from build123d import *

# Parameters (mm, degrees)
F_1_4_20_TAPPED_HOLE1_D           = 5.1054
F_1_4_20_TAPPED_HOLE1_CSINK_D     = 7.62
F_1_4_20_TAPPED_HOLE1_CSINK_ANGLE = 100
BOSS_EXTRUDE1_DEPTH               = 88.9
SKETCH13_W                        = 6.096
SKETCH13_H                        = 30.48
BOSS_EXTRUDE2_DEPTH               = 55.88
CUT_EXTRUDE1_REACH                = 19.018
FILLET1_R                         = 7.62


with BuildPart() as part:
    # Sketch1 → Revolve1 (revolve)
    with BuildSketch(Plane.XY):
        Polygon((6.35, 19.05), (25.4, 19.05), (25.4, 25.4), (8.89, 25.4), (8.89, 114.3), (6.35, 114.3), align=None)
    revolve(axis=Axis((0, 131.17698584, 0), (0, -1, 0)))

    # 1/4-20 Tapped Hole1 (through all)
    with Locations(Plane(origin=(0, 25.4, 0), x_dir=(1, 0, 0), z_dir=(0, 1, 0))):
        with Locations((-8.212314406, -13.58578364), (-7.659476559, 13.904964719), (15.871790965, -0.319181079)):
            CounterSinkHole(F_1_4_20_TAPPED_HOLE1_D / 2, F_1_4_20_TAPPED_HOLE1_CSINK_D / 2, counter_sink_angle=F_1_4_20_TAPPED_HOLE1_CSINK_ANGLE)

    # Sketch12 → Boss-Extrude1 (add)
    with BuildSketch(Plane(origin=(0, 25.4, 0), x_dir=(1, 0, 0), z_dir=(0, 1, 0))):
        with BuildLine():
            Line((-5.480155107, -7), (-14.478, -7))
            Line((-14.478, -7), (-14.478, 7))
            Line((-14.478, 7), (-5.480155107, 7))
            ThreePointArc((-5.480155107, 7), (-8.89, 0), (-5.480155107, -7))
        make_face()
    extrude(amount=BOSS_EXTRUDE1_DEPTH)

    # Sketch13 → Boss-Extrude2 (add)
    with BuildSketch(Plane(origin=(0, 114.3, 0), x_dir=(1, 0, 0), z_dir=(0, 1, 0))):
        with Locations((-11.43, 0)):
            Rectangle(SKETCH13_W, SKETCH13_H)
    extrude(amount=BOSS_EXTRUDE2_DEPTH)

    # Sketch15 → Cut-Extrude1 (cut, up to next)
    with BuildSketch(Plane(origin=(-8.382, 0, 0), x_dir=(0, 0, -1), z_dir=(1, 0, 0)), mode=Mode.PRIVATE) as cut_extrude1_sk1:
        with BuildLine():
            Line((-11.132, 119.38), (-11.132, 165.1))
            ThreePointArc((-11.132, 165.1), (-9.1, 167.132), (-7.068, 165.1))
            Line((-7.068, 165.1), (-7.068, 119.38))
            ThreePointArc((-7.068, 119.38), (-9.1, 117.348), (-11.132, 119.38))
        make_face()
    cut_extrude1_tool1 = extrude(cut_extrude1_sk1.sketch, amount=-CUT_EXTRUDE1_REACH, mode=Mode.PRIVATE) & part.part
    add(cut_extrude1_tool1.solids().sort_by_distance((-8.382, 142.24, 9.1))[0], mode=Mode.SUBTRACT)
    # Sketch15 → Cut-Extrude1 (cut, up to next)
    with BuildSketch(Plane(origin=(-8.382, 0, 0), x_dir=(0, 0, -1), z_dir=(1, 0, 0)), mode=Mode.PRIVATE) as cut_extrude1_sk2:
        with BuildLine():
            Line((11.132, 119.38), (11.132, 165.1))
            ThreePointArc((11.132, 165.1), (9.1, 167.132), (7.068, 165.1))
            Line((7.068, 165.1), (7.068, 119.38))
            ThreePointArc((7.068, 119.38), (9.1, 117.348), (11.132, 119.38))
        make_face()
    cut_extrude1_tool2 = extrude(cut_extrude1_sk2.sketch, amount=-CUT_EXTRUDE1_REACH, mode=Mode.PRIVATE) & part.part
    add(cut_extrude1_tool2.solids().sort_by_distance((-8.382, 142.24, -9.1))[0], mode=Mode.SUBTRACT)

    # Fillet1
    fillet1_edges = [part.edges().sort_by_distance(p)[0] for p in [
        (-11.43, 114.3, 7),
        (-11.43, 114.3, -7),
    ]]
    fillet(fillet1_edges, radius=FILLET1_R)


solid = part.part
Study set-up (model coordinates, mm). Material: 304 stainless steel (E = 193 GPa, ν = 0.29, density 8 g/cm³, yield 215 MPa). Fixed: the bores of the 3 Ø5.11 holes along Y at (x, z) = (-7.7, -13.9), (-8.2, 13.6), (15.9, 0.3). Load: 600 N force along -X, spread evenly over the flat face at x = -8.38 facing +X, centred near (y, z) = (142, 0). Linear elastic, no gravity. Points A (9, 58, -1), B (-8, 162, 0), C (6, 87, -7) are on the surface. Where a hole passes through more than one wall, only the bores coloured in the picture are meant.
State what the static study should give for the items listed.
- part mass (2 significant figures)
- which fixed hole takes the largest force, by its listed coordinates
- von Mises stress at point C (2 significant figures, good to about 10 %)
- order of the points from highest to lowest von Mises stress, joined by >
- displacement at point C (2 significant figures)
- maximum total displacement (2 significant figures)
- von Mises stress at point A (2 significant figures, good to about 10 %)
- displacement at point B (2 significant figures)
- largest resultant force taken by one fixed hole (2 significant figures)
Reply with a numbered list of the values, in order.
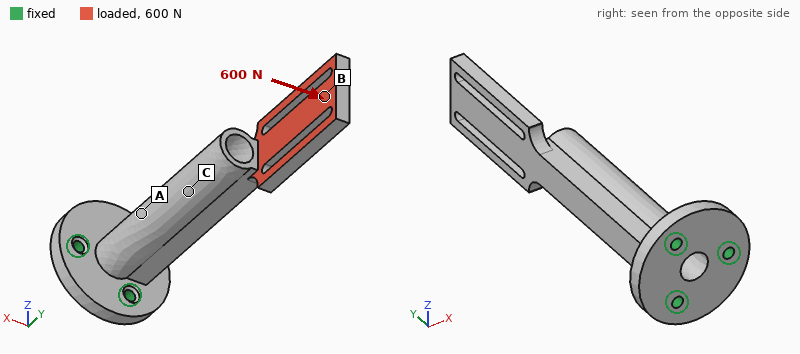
1. 310 g
2. (15.9, 0.3)
3. 34 MPa
4. A > C > B
5. 0.10 mm
6. 0.56 mm
7. 64 MPa
8. 0.49 mm
9. 2.7 kN
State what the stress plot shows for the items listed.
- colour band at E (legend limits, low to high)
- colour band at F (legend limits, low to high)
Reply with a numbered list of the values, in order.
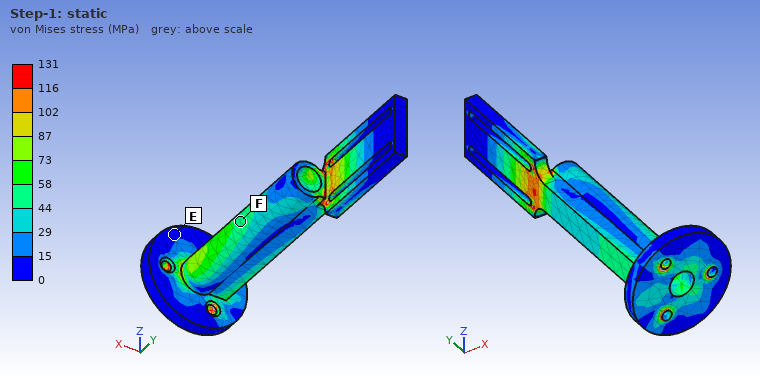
1. 0 to 15 MPa
2. 44 to 58 MPa
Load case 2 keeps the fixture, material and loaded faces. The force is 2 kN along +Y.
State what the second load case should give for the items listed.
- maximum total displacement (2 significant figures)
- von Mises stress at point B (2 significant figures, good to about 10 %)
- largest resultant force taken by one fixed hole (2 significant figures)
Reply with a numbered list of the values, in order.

1. 59 µm
2. 9.0 MPa
3. 1000 N
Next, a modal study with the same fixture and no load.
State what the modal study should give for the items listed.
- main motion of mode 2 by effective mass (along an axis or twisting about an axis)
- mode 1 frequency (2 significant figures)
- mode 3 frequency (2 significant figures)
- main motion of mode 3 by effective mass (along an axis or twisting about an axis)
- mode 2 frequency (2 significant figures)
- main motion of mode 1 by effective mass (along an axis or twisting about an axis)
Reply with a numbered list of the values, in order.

1. along X
2. 660 Hz
3. 2100 Hz
4. along X
5. 730 Hz
6. along Z
